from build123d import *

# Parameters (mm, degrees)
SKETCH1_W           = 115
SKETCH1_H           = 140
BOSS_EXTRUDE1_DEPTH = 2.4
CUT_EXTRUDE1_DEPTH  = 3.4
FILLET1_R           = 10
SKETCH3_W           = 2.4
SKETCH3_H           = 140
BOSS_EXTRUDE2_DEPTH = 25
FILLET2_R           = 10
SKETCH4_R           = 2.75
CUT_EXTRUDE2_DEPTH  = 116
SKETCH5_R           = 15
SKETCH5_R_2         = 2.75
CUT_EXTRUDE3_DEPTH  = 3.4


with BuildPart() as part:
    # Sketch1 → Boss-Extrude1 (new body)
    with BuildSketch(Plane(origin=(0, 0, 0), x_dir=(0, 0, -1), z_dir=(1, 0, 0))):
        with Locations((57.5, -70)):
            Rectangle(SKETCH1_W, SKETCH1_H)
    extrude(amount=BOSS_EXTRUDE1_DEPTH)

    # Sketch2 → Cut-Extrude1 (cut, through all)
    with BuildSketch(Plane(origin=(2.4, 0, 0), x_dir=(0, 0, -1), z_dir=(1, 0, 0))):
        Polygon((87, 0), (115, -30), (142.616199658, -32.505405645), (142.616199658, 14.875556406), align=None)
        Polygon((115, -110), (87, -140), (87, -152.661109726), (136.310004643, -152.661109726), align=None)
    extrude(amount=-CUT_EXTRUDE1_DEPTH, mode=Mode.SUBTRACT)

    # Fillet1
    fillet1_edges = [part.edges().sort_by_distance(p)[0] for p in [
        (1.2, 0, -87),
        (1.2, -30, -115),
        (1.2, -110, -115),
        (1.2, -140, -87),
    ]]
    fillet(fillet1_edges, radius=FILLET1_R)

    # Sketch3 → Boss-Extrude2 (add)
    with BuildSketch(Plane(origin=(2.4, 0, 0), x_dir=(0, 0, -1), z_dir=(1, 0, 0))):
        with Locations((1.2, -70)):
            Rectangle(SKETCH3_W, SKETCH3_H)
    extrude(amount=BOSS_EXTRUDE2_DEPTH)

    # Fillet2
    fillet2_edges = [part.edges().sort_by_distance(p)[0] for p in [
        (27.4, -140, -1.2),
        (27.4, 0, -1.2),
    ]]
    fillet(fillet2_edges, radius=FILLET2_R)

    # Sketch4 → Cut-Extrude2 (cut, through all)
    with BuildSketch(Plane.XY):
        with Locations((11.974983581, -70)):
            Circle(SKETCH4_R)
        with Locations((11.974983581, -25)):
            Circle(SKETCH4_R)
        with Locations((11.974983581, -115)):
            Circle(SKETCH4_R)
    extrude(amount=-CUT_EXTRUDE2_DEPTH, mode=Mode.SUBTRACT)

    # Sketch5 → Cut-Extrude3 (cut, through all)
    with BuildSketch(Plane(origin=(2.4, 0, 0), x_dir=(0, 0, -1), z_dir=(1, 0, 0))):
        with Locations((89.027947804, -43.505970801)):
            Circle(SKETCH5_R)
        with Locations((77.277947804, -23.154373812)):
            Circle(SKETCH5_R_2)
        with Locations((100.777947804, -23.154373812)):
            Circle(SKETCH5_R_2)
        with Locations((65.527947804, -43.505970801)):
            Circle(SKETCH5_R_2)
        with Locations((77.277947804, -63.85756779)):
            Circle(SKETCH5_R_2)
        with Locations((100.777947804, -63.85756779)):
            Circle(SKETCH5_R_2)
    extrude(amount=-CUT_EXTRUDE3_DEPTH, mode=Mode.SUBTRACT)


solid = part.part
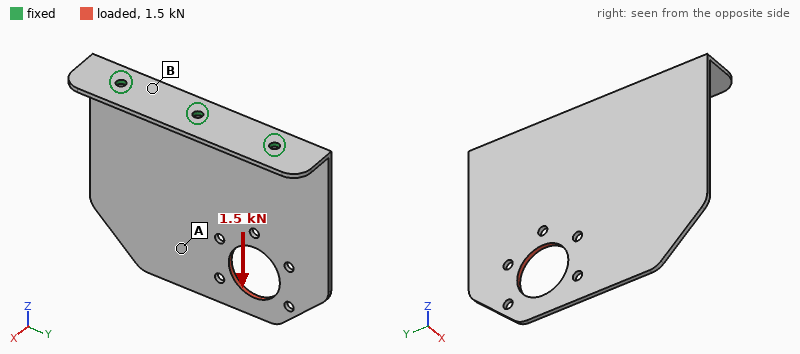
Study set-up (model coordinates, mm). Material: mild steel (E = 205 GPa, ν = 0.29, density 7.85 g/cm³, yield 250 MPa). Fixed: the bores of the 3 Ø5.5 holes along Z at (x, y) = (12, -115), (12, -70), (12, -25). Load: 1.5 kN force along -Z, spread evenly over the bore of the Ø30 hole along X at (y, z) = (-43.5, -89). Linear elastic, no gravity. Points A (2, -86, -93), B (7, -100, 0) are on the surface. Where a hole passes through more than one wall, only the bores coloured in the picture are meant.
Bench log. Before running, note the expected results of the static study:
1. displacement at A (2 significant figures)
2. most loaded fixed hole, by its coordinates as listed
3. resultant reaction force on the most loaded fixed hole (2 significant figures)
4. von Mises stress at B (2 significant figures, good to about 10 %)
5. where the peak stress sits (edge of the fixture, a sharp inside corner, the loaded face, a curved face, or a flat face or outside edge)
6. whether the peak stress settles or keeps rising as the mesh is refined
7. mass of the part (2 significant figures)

0.25 mm
(12, -25)
930 N
22 MPa
edge of the fixture
keeps rising
340 g
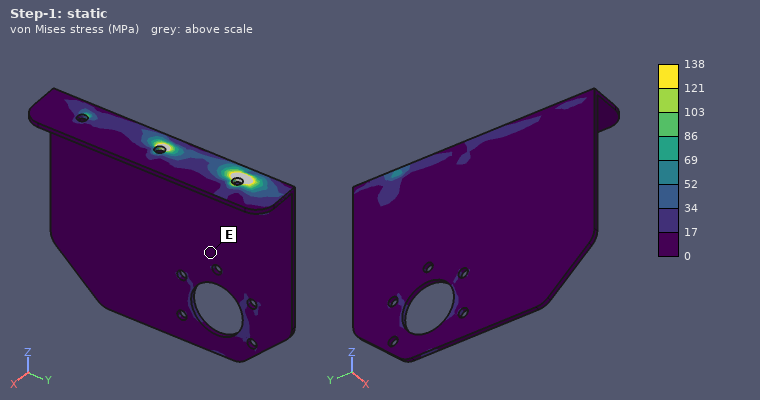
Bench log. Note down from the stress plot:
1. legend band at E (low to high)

0 to 17 MPa
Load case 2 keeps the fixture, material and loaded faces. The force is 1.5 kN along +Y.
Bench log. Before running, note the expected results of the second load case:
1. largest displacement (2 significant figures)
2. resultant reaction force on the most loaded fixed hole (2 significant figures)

0.31 mm
1.5 kN
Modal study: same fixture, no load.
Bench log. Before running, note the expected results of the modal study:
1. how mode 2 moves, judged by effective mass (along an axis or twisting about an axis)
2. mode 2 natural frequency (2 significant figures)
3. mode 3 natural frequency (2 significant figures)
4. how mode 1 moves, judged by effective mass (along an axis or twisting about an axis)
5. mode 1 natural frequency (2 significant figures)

twisting about Z
360 Hz
800 Hz
along X
150 Hz
